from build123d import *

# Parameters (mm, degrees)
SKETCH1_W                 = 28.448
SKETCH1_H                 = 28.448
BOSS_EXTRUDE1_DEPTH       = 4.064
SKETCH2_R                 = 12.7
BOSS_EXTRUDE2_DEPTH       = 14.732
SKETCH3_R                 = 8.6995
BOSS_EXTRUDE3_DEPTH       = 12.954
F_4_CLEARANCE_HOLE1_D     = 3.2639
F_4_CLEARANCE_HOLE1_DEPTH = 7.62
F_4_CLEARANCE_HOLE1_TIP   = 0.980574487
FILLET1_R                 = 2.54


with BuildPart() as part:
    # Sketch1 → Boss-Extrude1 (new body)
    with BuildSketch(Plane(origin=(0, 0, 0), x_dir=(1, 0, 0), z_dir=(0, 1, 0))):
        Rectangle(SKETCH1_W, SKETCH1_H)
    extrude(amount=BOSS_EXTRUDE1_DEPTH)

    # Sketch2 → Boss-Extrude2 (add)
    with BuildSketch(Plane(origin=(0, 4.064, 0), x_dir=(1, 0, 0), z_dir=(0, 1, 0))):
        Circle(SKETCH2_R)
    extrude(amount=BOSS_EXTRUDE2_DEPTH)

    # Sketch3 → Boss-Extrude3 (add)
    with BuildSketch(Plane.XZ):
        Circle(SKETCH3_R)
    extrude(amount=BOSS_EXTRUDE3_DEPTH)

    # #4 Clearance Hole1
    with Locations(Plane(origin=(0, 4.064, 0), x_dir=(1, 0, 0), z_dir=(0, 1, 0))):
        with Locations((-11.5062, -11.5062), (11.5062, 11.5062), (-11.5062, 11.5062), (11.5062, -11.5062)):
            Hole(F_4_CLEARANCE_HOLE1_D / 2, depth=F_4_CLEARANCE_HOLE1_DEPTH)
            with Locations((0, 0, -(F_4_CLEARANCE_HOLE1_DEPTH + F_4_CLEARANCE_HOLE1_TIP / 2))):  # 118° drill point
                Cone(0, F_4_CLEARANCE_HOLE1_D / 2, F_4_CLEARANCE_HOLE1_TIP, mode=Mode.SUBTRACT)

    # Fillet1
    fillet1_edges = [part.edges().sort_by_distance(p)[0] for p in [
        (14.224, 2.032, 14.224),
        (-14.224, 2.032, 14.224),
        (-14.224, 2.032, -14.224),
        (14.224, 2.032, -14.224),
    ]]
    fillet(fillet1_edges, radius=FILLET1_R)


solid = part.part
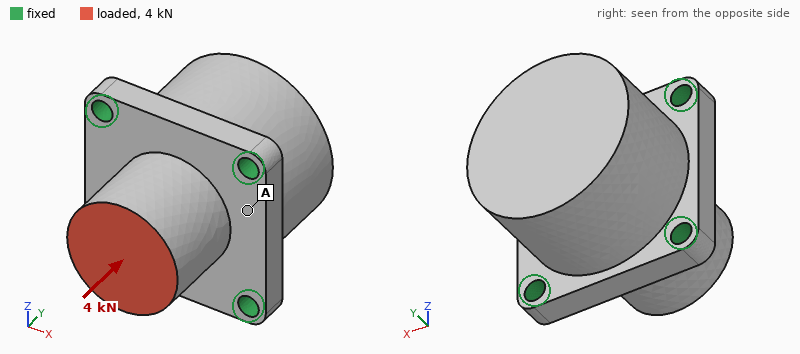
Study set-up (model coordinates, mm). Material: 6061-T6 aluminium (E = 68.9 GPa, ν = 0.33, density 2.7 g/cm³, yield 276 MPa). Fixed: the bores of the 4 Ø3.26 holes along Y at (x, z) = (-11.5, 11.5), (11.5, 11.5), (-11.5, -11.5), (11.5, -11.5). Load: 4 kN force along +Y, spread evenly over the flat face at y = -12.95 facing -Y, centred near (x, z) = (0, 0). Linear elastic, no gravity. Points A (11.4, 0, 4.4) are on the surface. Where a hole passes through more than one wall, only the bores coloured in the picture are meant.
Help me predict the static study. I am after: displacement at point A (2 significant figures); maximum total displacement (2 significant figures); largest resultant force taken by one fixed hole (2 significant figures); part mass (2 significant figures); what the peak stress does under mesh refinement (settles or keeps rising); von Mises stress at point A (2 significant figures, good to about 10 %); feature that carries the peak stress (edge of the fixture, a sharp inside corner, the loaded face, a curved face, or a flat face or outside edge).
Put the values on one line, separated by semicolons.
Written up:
7.6 µm; 13 µm; 1.0 kN; 37 g; keeps rising; 25 MPa; edge of the fixture
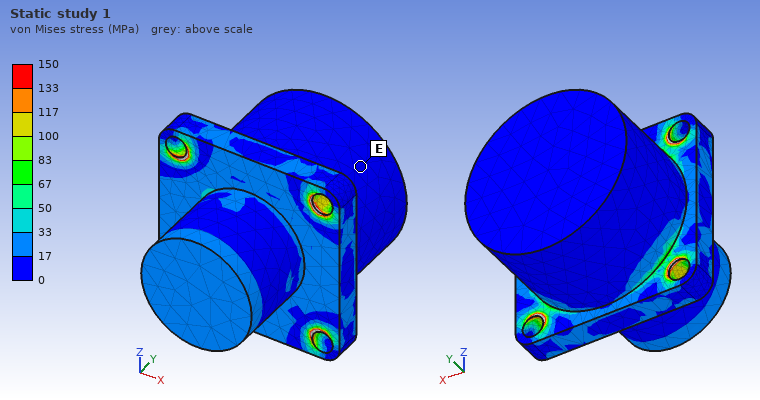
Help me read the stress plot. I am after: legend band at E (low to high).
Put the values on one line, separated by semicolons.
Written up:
0 to 17 MPa
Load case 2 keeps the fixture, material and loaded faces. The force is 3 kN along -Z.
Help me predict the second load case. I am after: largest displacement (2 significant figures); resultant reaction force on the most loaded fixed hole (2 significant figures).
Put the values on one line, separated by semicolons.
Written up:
46 µm; 1.3 kN
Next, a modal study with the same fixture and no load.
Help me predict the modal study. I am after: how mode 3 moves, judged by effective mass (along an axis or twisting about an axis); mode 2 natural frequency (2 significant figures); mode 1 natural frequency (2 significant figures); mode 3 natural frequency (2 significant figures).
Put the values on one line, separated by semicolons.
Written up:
along Y; 16 kHz; 16 kHz; 18 kHz
